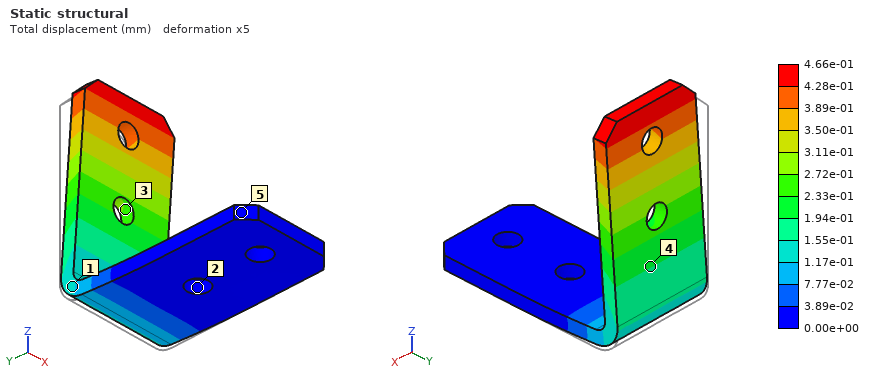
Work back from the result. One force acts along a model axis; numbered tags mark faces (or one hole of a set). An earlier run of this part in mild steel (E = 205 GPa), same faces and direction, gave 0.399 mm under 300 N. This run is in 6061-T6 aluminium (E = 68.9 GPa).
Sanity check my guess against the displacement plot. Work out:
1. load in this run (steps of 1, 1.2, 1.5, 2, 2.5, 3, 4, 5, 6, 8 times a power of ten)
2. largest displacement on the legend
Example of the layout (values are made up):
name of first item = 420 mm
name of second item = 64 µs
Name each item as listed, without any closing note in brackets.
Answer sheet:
load in this run = 120 N
largest displacement on the legend = 4.66e-01 mm
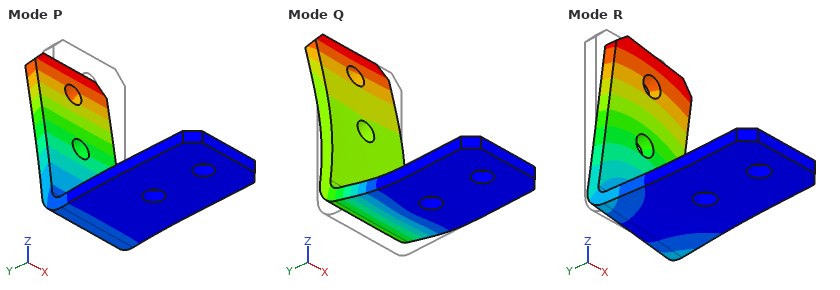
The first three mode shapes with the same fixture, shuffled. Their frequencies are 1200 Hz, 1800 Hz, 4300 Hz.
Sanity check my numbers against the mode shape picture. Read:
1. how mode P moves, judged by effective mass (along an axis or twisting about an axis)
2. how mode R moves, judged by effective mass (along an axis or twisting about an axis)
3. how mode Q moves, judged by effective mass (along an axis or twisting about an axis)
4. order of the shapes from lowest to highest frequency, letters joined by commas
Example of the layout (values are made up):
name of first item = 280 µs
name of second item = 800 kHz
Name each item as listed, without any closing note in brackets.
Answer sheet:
how mode P moves, judged by effective mass = along Y
how mode R moves, judged by effective mass = along X
how mode Q moves, judged by effective mass = along Z
order of the shapes from lowest to highest frequency, letters joined by commas = P, R, Q
